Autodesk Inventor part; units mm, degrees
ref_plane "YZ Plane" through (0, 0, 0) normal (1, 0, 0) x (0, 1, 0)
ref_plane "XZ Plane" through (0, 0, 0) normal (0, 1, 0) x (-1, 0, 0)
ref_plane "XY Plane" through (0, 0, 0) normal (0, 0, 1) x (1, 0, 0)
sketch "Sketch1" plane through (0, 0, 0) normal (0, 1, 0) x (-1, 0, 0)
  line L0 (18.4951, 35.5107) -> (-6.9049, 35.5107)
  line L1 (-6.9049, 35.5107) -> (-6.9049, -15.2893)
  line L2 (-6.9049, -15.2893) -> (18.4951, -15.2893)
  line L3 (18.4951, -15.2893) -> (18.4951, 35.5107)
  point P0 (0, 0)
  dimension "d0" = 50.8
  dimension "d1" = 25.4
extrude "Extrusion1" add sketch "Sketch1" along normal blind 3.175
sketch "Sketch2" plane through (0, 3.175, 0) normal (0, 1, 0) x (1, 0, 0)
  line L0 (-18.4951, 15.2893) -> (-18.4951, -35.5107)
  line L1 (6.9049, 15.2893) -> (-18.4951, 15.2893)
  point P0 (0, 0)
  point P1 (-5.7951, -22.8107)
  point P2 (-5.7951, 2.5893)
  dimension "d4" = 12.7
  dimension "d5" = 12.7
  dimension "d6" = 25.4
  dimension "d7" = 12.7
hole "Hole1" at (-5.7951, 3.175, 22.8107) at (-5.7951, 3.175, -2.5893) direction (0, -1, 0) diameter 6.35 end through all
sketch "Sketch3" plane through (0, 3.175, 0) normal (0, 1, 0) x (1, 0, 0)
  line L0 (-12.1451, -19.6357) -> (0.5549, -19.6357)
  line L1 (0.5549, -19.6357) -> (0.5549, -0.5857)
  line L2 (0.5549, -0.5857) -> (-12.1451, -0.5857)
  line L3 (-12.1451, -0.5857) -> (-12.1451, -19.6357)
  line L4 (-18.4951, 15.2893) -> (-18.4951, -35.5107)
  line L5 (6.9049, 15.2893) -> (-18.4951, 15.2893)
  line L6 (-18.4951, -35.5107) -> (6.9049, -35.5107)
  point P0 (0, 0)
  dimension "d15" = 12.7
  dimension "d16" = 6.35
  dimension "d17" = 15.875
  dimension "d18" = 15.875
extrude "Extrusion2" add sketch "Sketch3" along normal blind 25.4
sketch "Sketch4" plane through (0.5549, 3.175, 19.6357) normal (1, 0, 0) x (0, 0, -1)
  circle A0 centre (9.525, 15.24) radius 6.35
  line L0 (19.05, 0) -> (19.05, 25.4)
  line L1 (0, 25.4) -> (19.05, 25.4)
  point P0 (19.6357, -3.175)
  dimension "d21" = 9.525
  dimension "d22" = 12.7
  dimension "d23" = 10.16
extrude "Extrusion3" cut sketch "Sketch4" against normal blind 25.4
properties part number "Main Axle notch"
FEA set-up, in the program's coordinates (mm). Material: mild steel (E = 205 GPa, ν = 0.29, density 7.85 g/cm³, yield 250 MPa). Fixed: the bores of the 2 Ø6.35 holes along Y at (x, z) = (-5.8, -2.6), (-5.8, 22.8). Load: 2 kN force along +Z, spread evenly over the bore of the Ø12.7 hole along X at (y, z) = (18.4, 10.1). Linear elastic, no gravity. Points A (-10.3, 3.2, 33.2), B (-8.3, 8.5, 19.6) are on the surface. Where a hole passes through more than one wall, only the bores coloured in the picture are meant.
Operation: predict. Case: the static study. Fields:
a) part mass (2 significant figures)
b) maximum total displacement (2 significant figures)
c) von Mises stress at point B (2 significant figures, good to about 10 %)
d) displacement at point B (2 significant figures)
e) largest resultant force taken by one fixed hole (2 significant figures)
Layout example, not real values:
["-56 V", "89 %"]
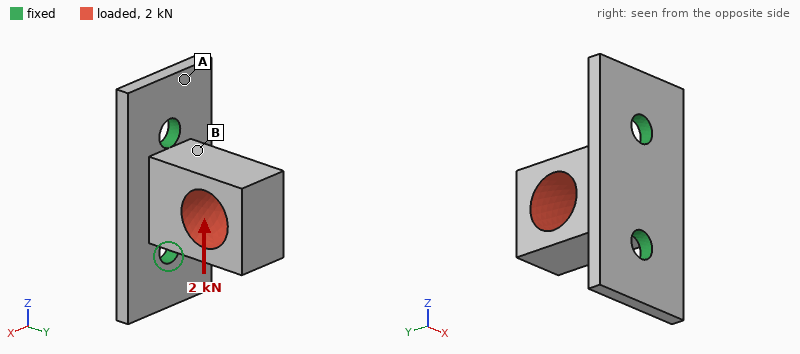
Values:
["66 g", "18 µm", "46 MPa", "3.4 µm", "2.0 kN"]
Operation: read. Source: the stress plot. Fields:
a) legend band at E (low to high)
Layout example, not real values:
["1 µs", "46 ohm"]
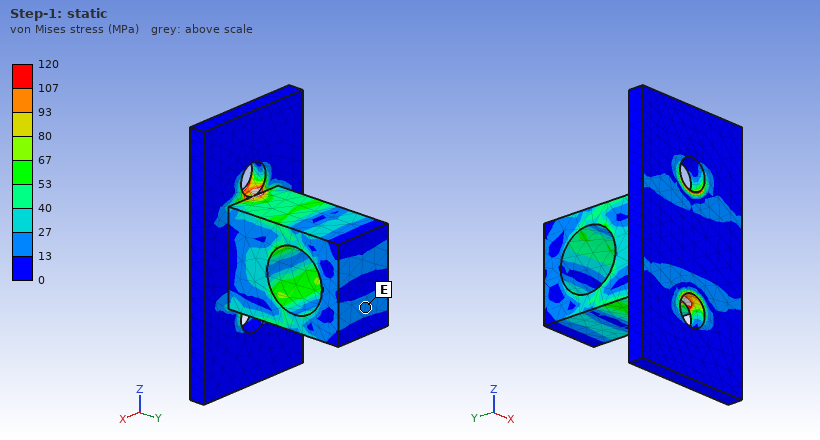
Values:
["13 to 27 MPa"]
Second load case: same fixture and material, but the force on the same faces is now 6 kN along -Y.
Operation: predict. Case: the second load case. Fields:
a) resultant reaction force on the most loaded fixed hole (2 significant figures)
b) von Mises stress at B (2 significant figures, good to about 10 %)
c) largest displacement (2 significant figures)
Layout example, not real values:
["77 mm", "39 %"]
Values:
["3.2 kN", "66 MPa", "11 µm"]
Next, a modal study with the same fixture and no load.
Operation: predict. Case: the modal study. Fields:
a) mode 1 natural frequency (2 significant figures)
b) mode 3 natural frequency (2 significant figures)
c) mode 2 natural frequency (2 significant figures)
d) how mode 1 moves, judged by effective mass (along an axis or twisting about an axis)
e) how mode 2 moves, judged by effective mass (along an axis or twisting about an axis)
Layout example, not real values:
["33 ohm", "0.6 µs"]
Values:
["6200 Hz", "17 kHz", "12 kHz", "along X", "along Z"]
